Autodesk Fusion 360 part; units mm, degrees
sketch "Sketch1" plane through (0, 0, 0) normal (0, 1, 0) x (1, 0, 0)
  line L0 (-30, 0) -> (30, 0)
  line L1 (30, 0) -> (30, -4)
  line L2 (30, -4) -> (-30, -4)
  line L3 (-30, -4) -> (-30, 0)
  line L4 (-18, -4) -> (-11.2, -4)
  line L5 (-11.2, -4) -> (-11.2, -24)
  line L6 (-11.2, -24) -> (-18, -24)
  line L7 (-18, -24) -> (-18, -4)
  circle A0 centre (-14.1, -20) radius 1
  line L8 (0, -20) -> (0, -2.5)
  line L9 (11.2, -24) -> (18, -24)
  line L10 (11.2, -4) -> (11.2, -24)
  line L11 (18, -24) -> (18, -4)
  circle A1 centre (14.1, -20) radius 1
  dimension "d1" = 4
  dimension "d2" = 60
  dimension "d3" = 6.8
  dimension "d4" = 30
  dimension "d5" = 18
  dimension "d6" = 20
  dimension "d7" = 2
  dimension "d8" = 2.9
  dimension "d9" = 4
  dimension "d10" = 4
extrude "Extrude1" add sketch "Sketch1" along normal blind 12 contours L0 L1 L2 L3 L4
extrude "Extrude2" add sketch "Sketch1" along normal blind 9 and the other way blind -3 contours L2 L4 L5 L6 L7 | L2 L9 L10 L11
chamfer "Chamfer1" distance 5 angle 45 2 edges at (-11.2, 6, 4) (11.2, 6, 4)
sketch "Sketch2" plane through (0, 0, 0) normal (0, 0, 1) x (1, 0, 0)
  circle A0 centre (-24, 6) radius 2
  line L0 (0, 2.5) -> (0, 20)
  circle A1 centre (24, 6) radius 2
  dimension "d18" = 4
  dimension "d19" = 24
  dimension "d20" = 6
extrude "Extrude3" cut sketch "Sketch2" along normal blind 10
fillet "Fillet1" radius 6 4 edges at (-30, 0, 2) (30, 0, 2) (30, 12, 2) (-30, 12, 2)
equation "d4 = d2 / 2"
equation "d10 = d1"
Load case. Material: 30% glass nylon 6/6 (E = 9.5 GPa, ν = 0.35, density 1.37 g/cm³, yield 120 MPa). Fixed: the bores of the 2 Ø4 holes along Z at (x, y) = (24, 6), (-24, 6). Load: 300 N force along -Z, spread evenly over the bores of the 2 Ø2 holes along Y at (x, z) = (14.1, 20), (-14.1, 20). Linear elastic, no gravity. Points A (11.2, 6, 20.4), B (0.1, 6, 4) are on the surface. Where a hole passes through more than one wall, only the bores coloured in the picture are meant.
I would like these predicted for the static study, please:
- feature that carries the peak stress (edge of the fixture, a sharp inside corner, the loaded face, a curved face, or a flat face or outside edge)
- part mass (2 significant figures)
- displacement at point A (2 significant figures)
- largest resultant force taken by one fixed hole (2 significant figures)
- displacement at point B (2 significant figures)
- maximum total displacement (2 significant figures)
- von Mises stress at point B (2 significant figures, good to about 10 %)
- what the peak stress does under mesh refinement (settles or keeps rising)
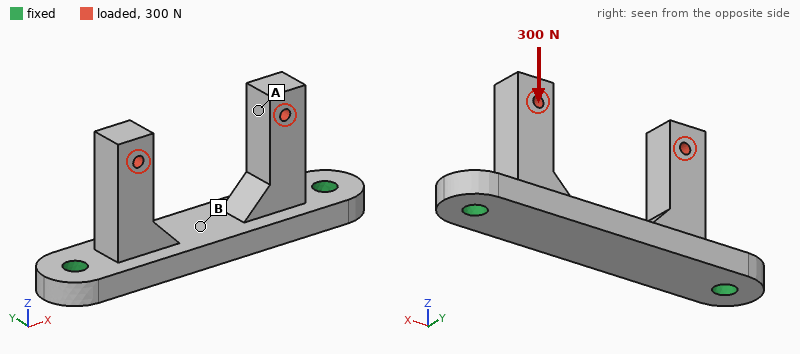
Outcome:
edge of the fixture
6.0 g
0.12 mm
150 N
0.095 mm
0.14 mm
12 MPa
keeps rising
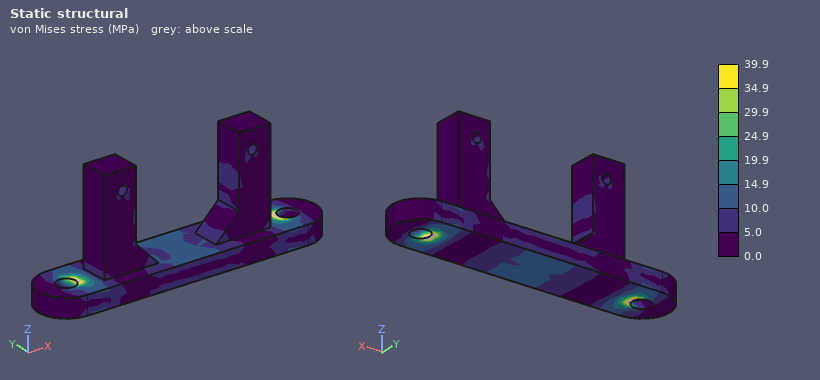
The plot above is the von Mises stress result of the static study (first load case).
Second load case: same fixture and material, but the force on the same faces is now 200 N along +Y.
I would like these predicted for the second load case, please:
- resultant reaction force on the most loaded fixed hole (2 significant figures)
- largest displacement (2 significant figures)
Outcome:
100 N
0.52 mm
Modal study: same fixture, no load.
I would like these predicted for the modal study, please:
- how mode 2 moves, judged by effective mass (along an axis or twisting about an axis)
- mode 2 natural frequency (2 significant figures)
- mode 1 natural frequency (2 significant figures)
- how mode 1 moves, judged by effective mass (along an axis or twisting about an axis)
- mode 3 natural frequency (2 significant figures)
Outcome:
along Y
3200 Hz
3100 Hz
along Z
4000 Hz
